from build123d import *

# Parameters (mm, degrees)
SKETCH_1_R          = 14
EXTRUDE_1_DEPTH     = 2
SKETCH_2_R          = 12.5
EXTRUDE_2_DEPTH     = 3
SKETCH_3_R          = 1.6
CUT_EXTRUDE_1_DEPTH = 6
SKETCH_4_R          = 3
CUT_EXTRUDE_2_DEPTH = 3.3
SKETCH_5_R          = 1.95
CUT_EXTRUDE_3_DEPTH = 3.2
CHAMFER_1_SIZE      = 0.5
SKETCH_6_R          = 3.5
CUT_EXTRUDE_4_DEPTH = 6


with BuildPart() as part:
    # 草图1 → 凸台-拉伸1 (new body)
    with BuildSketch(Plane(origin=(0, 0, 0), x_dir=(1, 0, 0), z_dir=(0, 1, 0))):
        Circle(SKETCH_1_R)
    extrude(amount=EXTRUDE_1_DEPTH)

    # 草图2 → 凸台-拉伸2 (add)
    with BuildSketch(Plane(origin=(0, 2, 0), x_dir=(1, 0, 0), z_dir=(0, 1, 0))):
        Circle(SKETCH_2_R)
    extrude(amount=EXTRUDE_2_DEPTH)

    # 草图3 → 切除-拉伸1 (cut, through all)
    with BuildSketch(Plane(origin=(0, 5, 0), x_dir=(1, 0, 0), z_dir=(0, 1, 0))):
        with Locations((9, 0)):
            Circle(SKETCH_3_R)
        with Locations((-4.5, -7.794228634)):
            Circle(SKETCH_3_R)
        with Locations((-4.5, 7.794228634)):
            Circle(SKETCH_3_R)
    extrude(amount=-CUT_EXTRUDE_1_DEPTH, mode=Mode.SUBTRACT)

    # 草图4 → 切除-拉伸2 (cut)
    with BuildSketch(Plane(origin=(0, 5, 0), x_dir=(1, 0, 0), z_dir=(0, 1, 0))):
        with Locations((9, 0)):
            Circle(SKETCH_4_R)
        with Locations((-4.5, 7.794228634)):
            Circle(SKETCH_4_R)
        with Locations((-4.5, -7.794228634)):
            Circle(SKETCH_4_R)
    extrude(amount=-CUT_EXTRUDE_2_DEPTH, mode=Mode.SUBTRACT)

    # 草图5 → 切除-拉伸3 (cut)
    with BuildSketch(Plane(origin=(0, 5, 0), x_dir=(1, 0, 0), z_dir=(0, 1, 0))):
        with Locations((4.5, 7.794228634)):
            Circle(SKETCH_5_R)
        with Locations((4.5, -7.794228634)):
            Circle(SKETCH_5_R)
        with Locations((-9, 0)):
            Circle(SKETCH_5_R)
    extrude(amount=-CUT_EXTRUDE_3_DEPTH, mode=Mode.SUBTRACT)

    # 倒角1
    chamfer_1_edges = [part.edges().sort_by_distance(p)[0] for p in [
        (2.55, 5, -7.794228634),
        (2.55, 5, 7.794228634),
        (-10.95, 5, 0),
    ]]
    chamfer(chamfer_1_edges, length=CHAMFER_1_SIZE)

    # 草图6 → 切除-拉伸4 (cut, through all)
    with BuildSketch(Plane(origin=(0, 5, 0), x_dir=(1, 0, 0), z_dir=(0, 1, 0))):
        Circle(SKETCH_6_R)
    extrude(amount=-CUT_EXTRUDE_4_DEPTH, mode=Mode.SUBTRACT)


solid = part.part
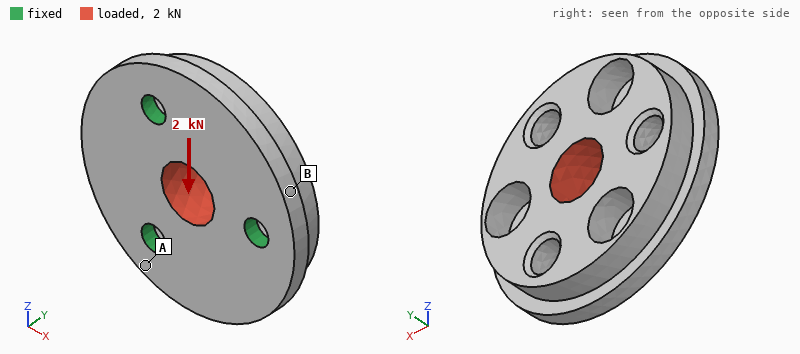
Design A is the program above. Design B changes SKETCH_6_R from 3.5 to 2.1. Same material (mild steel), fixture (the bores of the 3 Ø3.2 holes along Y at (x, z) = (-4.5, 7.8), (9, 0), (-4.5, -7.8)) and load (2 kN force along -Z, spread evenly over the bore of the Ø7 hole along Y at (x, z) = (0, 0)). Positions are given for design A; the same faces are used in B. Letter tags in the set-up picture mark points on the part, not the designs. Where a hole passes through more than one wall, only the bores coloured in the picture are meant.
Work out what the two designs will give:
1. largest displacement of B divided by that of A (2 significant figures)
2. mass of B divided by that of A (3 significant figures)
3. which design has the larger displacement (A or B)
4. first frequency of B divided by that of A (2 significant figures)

0.88
1.06
A
1.0
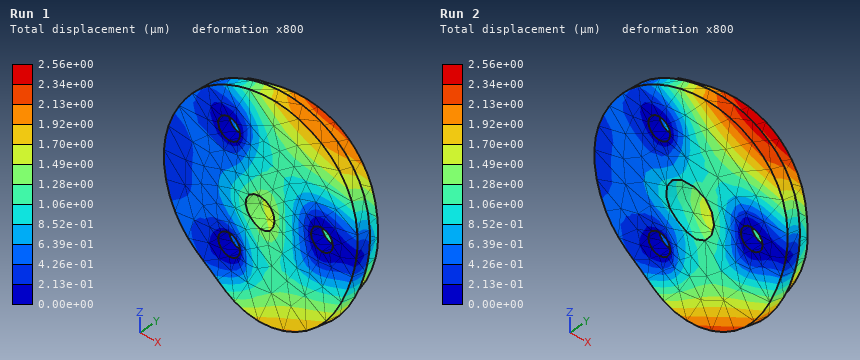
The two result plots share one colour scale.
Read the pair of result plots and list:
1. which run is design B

Run 1
